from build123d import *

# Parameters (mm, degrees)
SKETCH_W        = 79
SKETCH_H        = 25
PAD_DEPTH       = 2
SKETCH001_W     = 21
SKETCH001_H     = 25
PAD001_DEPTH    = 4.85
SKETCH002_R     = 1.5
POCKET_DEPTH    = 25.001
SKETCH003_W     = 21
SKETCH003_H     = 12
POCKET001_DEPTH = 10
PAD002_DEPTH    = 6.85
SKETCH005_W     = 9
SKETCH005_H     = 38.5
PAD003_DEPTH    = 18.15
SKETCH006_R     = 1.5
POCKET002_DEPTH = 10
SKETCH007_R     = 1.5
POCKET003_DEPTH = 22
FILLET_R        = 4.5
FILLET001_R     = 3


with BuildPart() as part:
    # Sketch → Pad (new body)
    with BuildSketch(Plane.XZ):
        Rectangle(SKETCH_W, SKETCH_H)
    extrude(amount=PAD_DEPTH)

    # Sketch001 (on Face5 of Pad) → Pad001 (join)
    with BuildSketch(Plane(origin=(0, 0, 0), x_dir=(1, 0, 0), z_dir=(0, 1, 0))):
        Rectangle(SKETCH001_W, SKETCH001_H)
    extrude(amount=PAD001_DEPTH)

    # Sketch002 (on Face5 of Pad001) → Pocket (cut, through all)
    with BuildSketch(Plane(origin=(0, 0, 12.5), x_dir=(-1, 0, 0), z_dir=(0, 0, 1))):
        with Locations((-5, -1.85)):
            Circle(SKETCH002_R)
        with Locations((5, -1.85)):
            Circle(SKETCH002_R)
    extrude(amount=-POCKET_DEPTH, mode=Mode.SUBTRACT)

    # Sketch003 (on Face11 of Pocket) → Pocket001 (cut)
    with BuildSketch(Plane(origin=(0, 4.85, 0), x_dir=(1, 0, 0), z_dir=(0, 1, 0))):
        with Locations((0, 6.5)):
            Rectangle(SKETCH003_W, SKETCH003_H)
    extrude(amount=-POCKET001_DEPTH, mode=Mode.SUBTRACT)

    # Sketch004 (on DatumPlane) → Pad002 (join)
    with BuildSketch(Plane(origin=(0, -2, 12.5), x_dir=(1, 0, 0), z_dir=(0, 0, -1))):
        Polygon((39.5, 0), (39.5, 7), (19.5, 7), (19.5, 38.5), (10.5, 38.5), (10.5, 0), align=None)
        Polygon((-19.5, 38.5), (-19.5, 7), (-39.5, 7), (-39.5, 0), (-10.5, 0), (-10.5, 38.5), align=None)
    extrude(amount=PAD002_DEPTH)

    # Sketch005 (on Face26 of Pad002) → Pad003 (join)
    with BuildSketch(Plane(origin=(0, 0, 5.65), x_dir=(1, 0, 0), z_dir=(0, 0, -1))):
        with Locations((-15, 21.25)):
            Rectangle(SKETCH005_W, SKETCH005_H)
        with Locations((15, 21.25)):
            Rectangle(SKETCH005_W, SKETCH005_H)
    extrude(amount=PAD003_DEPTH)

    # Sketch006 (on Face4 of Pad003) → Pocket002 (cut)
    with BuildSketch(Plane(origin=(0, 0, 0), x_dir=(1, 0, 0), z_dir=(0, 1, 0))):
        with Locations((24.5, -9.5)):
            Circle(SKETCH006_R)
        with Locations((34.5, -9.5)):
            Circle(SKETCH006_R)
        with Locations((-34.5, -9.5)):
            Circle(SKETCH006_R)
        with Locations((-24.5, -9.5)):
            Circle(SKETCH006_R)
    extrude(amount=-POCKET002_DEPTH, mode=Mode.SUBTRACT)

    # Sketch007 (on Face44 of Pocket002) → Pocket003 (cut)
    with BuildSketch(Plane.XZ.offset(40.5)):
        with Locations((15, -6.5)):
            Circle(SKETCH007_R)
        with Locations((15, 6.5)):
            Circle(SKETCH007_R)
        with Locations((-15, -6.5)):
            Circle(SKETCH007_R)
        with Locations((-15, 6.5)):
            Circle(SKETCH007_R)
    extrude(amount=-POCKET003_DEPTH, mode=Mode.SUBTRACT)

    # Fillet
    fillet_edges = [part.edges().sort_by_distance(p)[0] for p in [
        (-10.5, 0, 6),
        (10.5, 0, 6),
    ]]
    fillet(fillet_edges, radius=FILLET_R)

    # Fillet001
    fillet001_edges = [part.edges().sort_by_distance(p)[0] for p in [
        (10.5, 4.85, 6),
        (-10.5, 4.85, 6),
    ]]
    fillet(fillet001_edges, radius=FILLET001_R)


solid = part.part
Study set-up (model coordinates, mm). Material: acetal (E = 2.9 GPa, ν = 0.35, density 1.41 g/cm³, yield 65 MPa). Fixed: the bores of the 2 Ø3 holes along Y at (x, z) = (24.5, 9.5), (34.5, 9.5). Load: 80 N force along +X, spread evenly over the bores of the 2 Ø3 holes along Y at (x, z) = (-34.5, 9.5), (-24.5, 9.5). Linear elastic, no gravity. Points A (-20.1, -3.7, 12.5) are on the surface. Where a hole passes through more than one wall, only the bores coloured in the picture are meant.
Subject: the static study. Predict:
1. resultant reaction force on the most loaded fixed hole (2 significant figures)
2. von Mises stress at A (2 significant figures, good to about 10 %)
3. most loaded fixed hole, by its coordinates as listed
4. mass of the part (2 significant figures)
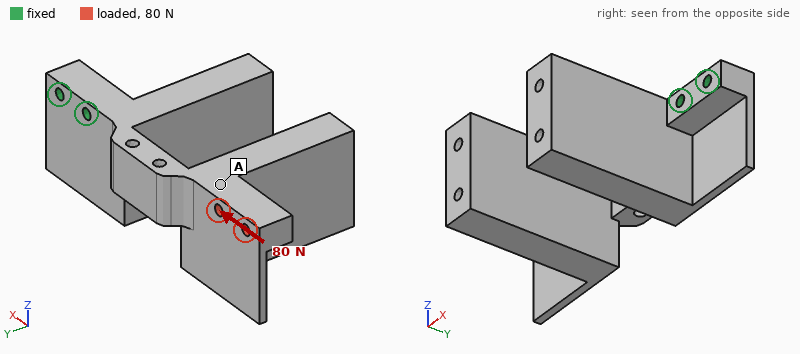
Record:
76 N
1.8 MPa
(24.5, 9.5)
32 g
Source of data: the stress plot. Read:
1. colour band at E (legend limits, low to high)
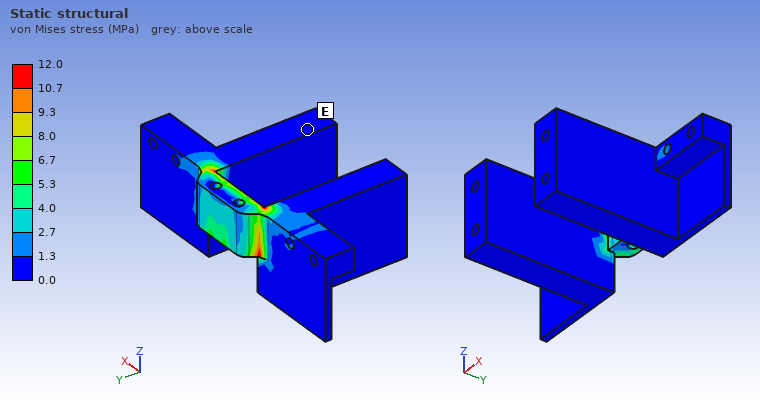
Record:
0.0 to 1.3 MPa
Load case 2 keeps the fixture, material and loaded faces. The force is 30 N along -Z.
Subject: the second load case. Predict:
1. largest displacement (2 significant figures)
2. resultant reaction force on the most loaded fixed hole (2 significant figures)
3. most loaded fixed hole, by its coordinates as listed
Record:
1.0 mm
140 N
(24.5, 9.5)
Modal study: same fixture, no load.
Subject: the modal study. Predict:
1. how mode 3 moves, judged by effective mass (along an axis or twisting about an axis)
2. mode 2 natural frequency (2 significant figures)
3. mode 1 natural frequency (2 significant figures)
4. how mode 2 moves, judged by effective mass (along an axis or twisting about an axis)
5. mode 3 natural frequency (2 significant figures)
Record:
along Y
230 Hz
160 Hz
along Z
480 Hz
